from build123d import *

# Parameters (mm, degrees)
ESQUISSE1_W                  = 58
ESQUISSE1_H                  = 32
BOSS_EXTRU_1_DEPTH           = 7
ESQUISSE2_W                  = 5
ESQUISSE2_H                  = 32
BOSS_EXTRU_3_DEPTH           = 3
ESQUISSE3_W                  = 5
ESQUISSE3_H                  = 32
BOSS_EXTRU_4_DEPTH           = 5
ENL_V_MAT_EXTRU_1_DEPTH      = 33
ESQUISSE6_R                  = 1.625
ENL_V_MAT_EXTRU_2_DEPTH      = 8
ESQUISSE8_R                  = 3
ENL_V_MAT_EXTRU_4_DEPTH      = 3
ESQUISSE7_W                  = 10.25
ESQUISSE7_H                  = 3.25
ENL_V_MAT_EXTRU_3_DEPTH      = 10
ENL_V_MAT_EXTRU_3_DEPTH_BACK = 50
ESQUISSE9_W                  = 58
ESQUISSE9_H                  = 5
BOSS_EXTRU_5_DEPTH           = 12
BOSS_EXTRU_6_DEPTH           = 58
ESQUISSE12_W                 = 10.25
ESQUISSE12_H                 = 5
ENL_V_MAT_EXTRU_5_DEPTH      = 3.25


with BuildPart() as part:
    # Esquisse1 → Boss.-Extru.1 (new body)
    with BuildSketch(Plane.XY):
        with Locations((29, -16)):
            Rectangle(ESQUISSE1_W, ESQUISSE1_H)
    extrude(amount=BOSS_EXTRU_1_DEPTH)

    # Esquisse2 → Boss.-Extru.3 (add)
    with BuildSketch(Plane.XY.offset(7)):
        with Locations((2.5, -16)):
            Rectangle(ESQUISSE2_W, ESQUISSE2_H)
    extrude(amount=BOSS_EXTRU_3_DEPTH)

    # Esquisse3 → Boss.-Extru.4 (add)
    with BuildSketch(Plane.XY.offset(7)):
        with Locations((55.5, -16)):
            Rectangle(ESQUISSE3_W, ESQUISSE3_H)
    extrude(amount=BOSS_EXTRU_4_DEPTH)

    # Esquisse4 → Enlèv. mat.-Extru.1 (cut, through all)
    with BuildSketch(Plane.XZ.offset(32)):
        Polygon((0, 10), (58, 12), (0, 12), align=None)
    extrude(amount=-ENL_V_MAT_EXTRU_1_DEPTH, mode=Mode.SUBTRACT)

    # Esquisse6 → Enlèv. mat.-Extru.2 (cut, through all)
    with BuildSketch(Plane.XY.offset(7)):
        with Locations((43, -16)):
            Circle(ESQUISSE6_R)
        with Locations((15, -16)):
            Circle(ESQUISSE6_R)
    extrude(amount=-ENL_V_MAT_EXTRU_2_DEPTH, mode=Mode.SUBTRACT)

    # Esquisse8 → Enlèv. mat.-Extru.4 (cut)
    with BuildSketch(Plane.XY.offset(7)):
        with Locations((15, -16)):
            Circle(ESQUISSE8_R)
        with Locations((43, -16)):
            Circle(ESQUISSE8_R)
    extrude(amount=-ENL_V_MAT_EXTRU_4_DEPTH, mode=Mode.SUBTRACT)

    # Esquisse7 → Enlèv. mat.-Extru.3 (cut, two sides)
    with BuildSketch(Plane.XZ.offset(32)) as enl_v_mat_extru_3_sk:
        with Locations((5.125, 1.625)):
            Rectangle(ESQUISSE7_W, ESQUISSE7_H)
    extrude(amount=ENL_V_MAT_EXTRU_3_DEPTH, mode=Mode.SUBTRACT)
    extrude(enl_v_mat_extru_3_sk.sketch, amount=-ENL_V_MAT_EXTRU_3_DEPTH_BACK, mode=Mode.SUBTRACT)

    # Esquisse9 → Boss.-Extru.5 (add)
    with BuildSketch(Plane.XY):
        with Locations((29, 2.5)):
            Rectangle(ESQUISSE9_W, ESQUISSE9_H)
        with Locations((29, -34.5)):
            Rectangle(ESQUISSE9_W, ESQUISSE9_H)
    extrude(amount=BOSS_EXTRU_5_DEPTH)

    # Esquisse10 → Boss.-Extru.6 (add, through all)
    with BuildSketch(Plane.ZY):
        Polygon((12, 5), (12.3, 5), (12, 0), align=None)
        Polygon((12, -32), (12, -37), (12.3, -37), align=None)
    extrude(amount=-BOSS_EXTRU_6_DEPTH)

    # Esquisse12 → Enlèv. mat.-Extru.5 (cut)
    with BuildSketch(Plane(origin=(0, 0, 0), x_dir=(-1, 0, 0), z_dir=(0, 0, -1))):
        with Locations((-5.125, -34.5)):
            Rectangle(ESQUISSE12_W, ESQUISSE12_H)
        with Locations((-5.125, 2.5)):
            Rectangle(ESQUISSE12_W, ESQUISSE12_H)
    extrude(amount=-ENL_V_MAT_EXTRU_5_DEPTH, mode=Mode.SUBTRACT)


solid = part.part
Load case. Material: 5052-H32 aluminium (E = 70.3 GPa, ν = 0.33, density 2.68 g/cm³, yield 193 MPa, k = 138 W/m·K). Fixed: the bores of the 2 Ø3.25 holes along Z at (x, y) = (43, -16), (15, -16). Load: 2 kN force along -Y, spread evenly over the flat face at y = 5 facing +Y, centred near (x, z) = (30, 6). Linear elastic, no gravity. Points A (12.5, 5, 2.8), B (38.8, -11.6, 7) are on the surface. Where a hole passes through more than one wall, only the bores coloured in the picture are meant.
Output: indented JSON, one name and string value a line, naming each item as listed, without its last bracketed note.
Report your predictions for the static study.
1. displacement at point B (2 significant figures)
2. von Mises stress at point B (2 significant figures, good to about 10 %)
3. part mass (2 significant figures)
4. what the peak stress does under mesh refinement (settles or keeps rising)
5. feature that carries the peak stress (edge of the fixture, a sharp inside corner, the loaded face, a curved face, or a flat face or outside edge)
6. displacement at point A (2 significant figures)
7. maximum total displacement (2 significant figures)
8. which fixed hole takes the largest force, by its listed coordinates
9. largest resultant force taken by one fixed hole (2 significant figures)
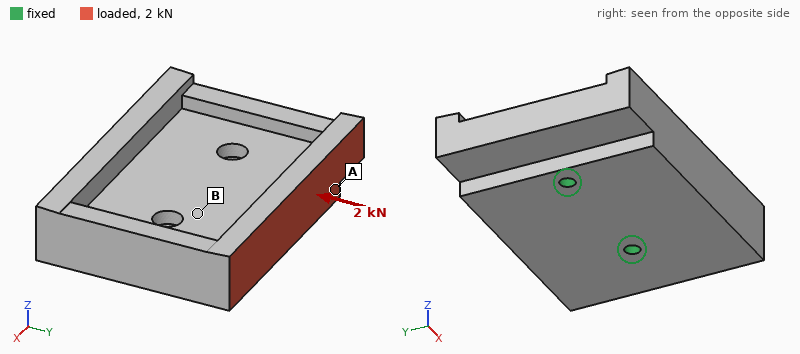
{
  "displacement at point B": "11 µm",
  "von Mises stress at point B": "16 MPa",
  "part mass": "53 g",
  "what the peak stress does under mesh refinement": "keeps rising",
  "feature that carries the peak stress": "edge of the fixture",
  "displacement at point A": "37 µm",
  "maximum total displacement": "45 µm",
  "which fixed hole takes the largest force, by its listed coordinates": "(43, -16)",
  "largest resultant force taken by one fixed hole": "1.1 kN"
}
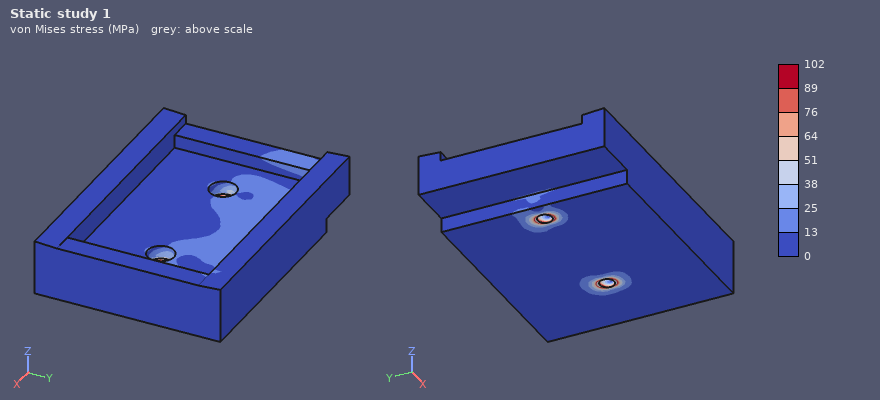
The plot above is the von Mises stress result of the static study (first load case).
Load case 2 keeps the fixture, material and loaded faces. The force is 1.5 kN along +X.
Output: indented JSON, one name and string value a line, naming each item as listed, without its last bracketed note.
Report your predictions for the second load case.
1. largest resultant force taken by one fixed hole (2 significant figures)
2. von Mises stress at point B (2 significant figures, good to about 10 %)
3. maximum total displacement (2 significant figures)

{
  "largest resultant force taken by one fixed hole": "1.4 kN",
  "von Mises stress at point B": "11 MPa",
  "maximum total displacement": "15 µm"
}
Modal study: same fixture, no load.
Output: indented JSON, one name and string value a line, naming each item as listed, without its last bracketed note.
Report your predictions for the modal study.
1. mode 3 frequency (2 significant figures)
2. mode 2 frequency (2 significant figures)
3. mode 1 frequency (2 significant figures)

{
  "mode 3 frequency": "9000 Hz",
  "mode 2 frequency": "8100 Hz",
  "mode 1 frequency": "3800 Hz"
}
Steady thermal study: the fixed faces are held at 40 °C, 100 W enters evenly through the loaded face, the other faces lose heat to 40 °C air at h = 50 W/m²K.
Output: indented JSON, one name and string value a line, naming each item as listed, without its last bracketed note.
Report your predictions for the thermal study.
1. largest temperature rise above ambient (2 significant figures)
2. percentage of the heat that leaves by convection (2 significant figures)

{
  "largest temperature rise above ambient": "52 K",
  "percentage of the heat that leaves by convection": "8.5 %"
}
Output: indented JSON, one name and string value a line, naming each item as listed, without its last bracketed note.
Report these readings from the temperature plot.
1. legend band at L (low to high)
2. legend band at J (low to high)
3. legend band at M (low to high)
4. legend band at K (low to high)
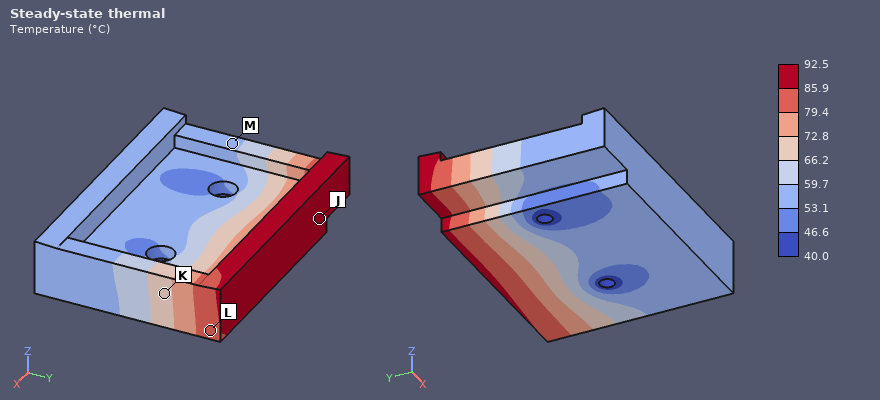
{
  "legend band at L": "79.4 to 85.9 °C",
  "legend band at J": "85.9 to 92.5 °C",
  "legend band at M": "53.1 to 59.7 °C",
  "legend band at K": "66.2 to 72.8 °C"
}
